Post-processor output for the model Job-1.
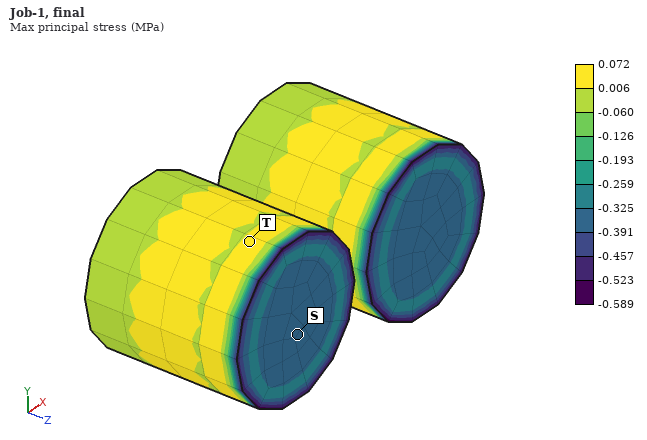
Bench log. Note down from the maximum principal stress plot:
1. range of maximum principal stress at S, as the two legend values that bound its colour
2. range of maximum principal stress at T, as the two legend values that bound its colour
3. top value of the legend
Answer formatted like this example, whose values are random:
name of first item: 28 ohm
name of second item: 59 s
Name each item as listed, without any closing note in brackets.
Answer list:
range of maximum principal stress at S, as the two legend values that bound its colour: -0.391 to -0.325 MPa
range of maximum principal stress at T, as the two legend values that bound its colour: 0.006 to 0.072 MPa
top value of the legend: 0.072 MPa
